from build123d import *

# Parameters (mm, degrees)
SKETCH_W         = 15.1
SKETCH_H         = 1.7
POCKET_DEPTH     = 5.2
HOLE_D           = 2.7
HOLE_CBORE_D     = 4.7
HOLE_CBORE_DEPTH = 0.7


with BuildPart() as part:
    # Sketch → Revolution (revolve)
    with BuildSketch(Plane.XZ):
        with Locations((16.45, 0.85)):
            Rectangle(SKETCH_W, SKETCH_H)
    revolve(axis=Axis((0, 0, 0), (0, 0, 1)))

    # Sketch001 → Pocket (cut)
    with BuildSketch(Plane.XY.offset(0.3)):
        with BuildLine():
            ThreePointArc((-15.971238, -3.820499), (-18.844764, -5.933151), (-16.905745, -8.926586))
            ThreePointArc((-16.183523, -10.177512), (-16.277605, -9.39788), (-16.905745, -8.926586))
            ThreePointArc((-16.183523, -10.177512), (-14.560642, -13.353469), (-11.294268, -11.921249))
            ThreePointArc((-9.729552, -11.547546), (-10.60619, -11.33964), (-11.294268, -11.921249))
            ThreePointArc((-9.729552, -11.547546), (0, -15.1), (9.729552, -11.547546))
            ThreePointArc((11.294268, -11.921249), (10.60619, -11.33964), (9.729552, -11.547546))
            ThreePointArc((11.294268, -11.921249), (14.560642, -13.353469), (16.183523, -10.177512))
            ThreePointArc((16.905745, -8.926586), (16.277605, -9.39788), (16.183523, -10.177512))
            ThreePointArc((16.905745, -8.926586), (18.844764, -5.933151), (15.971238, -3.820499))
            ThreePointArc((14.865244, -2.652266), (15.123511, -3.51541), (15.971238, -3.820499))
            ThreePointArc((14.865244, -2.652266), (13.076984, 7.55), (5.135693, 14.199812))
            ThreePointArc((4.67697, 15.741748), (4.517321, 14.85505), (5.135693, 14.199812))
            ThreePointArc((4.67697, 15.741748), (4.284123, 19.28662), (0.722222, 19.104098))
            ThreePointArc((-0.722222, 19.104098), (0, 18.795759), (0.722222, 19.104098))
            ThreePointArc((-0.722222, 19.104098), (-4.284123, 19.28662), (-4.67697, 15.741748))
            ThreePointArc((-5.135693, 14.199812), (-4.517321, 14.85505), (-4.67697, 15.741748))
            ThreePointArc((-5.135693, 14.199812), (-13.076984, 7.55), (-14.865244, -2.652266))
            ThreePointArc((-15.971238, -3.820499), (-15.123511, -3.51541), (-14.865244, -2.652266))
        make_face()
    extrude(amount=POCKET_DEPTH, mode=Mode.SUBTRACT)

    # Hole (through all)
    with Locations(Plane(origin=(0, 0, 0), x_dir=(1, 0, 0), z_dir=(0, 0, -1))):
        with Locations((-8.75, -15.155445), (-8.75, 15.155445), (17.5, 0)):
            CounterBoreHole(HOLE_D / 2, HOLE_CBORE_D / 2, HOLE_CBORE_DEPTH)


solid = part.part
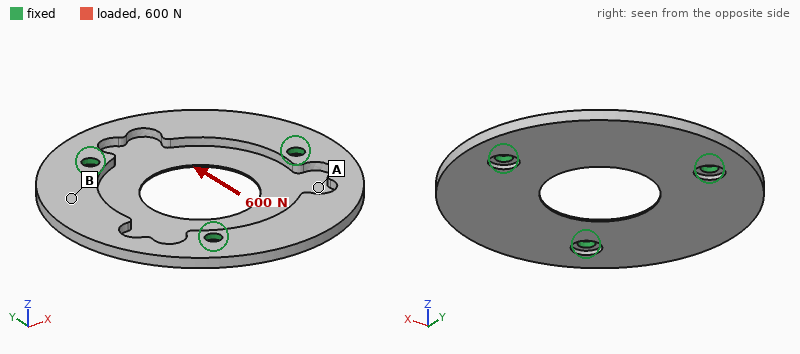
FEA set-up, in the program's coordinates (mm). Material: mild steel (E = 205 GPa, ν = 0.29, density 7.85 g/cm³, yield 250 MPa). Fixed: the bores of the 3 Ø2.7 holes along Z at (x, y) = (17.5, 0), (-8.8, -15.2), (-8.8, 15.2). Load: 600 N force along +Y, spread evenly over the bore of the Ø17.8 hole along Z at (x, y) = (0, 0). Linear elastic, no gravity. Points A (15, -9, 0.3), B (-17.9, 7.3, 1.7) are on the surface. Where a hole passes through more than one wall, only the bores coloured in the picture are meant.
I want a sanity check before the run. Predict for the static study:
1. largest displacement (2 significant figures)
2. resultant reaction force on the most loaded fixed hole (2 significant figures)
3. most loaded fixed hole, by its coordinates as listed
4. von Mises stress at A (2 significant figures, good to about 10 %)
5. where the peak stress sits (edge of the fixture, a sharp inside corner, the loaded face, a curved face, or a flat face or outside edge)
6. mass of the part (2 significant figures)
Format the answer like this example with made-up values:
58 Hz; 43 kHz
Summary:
13 µm; 230 N; (17.5, 0); 23 MPa; a curved face; 14 g
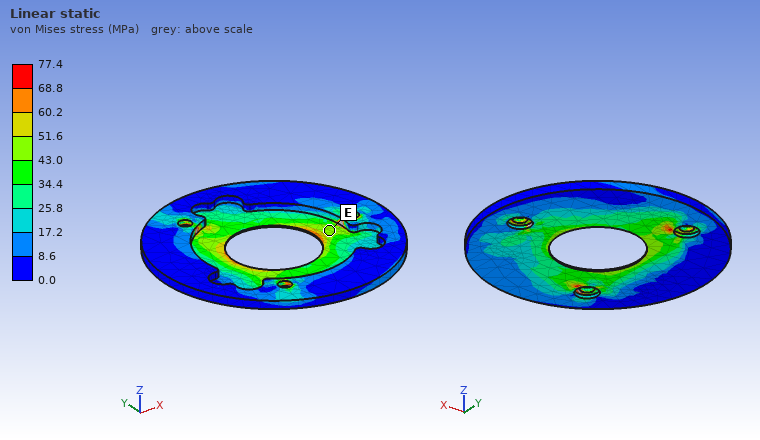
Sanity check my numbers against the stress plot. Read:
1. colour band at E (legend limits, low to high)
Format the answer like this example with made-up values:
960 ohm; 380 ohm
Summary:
43.0 to 51.6 MPa
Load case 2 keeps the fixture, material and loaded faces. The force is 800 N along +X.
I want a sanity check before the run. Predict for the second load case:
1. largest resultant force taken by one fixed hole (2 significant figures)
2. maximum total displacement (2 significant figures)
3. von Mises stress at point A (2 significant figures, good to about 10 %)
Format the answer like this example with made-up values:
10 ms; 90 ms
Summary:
290 N; 20 µm; 30 MPa
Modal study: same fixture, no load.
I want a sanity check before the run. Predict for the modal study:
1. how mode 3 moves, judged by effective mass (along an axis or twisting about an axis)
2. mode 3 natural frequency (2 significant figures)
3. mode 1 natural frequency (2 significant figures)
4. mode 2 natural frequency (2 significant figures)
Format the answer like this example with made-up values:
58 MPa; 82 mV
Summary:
along Z; 4400 Hz; 3800 Hz; 3800 Hz
